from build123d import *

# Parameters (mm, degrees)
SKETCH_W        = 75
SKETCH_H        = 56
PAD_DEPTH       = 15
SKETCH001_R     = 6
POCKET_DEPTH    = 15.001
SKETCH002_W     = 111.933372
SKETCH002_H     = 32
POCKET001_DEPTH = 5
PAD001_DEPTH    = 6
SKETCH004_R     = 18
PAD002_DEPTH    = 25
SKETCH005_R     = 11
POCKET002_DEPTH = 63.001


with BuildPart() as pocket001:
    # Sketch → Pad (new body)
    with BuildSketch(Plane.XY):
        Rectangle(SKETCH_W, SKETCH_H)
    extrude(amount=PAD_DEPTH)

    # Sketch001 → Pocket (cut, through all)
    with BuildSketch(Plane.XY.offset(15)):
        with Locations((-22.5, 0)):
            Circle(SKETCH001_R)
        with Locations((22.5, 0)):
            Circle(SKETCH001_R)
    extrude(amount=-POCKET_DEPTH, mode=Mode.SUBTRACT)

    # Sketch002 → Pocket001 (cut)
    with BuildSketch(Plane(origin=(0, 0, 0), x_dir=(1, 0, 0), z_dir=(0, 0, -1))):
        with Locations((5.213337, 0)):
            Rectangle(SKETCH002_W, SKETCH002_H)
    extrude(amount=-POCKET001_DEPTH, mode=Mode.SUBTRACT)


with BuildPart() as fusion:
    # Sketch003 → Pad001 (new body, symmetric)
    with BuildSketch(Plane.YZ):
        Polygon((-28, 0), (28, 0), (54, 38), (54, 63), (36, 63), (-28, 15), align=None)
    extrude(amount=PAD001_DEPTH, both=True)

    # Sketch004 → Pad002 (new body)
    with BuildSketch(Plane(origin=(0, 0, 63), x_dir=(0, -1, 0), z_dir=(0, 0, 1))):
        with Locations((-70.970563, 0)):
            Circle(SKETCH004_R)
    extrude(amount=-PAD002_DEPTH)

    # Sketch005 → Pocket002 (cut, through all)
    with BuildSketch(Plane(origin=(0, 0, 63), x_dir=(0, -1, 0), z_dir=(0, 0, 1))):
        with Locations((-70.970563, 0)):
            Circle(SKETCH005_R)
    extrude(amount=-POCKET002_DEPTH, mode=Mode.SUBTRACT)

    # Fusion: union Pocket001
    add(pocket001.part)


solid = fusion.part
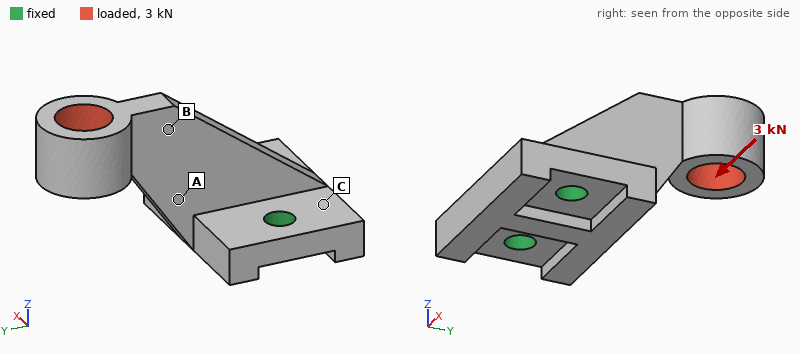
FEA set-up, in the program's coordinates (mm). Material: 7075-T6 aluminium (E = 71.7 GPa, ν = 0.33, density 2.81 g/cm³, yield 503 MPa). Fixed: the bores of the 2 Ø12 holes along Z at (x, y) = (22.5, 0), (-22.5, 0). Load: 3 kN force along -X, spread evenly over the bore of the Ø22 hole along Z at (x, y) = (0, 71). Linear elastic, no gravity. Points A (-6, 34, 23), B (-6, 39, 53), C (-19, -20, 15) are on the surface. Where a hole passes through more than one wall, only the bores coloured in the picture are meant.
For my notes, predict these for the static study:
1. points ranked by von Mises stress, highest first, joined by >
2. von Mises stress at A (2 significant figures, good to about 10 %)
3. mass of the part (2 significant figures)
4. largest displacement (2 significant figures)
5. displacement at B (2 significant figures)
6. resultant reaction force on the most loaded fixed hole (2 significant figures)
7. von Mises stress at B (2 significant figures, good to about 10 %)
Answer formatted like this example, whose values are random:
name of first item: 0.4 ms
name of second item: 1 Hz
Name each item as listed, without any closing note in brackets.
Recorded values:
points ranked by von Mises stress, highest first, joined by >: A > B > C
von Mises stress at A: 170 MPa
mass of the part: 260 g
largest displacement: 1.3 mm
displacement at B: 0.40 mm
resultant reaction force on the most loaded fixed hole: 5.4 kN
von Mises stress at B: 98 MPa
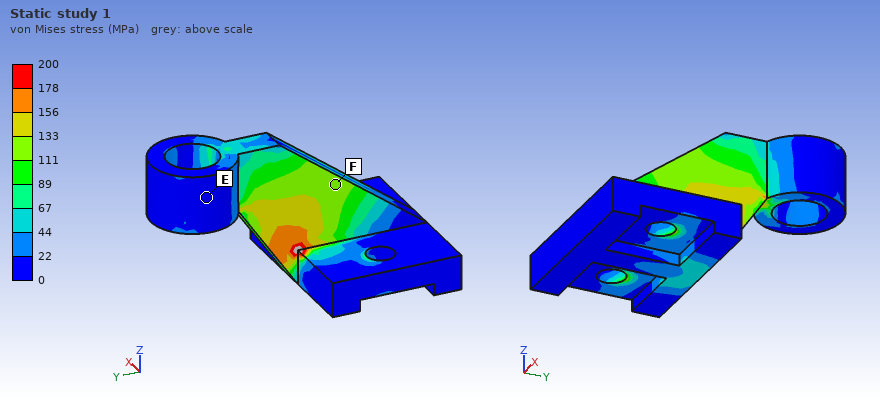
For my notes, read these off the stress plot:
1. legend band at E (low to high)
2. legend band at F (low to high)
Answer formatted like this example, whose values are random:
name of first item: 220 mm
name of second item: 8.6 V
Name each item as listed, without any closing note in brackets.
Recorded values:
legend band at E: 0 to 22 MPa
legend band at F: 111 to 133 MPa
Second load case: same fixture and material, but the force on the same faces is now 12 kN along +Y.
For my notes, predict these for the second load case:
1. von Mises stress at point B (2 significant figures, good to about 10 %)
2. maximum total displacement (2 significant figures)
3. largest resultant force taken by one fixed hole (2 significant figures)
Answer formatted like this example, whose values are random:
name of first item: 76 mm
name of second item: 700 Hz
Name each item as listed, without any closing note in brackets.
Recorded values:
von Mises stress at point B: 51 MPa
maximum total displacement: 0.86 mm
largest resultant force taken by one fixed hole: 6.0 kN
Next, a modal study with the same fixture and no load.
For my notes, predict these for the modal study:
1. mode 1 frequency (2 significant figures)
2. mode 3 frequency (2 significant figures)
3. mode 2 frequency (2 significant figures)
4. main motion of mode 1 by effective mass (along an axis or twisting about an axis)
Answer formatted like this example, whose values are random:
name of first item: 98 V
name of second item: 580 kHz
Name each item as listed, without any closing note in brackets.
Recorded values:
mode 1 frequency: 1200 Hz
mode 3 frequency: 3600 Hz
mode 2 frequency: 1800 Hz
main motion of mode 1 by effective mass: along X
